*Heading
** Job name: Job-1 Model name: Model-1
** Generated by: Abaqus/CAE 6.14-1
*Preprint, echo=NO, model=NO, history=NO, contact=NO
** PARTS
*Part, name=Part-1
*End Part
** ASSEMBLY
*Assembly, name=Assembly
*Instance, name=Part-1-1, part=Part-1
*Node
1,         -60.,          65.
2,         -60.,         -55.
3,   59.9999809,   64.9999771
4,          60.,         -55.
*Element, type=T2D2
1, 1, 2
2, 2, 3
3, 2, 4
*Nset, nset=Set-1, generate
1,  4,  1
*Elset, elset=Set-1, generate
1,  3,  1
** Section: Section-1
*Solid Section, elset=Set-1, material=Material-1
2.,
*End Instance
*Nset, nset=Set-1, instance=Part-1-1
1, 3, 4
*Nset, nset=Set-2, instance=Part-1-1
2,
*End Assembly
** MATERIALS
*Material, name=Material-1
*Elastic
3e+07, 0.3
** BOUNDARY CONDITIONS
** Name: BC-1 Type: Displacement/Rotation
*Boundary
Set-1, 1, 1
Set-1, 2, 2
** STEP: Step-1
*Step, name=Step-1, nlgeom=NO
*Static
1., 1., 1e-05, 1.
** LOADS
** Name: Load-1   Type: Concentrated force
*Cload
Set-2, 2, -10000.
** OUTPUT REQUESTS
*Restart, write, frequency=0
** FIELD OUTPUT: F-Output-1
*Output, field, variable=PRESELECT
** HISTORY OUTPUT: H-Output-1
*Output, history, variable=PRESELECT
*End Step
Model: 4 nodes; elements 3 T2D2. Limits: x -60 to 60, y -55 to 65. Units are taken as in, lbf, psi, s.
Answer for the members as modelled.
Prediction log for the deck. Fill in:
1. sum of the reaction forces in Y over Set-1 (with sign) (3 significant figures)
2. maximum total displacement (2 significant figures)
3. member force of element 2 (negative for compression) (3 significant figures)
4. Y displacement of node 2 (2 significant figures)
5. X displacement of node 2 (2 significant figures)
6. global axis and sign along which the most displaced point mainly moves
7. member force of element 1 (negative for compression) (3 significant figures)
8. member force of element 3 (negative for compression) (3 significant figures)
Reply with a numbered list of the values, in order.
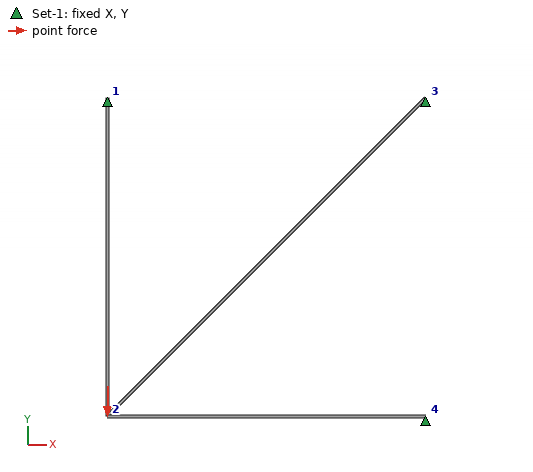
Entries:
1. 10000 lbf
2. 0.016 in
3. 2930 lbf
4. -0.016 in
5. 0.0041 in
6. -Y
7. 7930 lbf
8. -2070 lbf
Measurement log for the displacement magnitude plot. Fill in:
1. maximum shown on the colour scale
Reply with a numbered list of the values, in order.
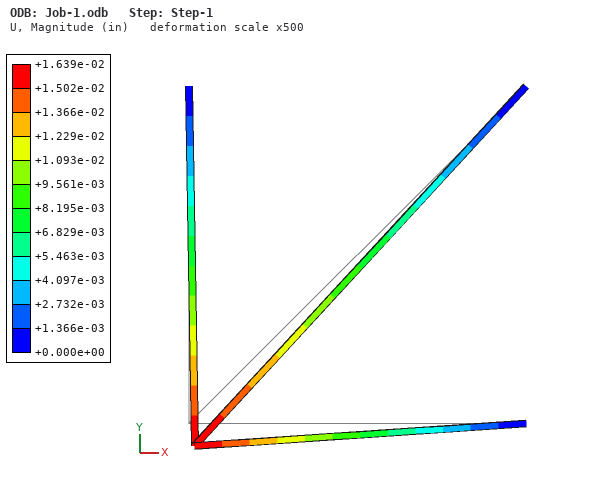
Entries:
1. +1.639e-02 in
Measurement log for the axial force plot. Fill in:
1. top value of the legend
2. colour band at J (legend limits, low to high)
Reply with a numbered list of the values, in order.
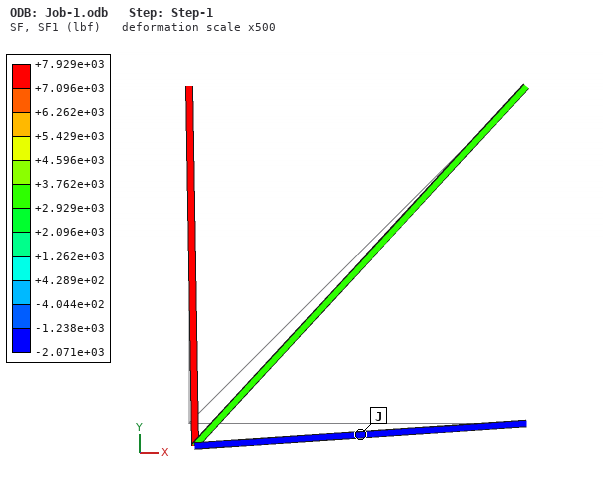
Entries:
1. +7.929e+03 lbf
2. -2.071e+03 to -1.238e+03 lbf
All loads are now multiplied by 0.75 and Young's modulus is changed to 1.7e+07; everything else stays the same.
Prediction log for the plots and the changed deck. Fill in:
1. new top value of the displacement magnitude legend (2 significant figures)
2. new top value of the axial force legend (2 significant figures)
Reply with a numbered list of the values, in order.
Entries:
1. 0.022 in
2. 5900 lbf
